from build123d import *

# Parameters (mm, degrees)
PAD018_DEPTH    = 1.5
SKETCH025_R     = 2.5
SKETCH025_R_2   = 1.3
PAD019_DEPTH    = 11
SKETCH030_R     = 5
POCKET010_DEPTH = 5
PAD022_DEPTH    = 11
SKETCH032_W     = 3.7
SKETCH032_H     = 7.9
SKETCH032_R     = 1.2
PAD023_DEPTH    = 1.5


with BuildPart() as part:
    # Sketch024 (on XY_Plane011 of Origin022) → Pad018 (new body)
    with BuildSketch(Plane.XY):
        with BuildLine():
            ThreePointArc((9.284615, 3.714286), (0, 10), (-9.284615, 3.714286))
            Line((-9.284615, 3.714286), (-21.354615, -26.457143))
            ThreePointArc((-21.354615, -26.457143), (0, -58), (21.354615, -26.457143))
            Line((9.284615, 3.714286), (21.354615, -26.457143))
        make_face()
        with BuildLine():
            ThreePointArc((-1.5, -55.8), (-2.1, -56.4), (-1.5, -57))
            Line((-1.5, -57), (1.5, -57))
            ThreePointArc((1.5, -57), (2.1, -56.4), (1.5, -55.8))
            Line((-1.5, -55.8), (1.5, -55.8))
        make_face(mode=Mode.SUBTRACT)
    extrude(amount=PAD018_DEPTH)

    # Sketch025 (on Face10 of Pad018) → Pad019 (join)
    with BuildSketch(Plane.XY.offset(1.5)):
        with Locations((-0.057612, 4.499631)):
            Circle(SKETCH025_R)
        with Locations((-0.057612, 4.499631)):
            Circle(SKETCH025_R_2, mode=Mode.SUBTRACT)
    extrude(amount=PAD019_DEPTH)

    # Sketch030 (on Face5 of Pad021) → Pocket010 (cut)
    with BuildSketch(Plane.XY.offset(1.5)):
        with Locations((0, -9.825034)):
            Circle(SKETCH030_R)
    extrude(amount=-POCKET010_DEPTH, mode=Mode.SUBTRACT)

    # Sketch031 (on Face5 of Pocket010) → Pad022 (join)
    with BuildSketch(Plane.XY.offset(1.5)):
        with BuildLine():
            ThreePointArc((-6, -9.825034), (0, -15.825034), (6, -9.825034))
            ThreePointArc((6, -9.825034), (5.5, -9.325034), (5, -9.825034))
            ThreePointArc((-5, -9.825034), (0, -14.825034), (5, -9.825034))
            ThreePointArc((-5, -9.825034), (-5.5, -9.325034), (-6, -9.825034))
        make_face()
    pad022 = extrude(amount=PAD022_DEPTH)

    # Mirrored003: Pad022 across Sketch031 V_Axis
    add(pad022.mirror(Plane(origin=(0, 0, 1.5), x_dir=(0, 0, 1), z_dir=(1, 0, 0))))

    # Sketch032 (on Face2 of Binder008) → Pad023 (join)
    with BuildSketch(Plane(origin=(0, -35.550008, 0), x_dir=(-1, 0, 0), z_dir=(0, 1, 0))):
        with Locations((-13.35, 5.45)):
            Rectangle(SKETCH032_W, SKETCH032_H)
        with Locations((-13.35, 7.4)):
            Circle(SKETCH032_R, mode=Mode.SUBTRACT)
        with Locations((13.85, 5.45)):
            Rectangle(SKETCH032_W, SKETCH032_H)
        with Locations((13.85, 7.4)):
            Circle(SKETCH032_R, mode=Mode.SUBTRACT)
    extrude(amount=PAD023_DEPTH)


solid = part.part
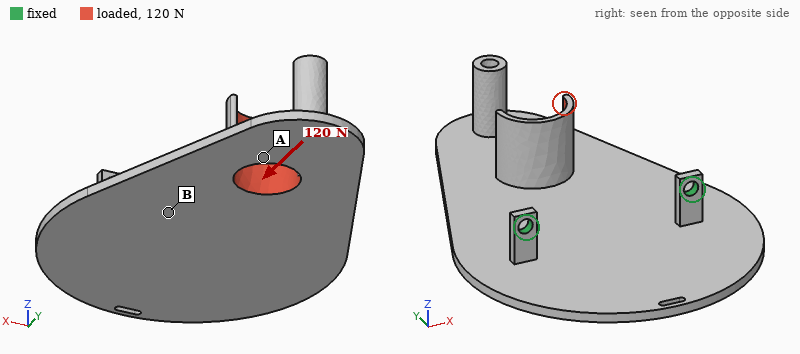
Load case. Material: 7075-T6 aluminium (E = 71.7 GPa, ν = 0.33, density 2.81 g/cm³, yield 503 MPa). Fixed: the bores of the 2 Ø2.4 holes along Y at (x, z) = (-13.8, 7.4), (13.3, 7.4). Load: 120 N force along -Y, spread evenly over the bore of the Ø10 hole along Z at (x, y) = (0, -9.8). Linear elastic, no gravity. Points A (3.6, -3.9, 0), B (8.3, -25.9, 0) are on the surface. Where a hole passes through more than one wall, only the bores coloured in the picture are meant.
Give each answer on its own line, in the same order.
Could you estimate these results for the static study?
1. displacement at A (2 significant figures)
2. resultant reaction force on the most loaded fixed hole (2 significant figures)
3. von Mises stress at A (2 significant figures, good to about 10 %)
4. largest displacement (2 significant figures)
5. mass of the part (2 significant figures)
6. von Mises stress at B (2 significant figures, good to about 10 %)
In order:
0.56 mm
61 N
12 MPa
0.89 mm
10 g
33 MPa
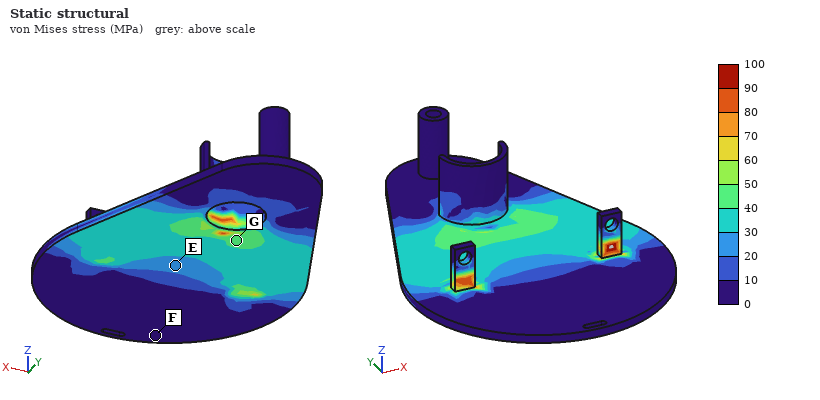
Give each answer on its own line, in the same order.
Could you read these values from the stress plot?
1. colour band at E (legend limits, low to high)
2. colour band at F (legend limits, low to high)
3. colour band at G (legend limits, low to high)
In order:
20 to 30 MPa
0 to 10 MPa
40 to 50 MPa
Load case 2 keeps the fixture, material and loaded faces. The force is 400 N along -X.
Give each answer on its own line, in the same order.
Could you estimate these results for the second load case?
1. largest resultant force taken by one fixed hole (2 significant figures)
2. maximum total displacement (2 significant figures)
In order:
380 N
0.89 mm
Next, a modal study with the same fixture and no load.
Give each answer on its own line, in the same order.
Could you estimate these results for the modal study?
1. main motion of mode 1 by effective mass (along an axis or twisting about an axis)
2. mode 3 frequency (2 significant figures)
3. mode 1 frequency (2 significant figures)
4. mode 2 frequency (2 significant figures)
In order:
along Z
1900 Hz
370 Hz
1700 Hz
